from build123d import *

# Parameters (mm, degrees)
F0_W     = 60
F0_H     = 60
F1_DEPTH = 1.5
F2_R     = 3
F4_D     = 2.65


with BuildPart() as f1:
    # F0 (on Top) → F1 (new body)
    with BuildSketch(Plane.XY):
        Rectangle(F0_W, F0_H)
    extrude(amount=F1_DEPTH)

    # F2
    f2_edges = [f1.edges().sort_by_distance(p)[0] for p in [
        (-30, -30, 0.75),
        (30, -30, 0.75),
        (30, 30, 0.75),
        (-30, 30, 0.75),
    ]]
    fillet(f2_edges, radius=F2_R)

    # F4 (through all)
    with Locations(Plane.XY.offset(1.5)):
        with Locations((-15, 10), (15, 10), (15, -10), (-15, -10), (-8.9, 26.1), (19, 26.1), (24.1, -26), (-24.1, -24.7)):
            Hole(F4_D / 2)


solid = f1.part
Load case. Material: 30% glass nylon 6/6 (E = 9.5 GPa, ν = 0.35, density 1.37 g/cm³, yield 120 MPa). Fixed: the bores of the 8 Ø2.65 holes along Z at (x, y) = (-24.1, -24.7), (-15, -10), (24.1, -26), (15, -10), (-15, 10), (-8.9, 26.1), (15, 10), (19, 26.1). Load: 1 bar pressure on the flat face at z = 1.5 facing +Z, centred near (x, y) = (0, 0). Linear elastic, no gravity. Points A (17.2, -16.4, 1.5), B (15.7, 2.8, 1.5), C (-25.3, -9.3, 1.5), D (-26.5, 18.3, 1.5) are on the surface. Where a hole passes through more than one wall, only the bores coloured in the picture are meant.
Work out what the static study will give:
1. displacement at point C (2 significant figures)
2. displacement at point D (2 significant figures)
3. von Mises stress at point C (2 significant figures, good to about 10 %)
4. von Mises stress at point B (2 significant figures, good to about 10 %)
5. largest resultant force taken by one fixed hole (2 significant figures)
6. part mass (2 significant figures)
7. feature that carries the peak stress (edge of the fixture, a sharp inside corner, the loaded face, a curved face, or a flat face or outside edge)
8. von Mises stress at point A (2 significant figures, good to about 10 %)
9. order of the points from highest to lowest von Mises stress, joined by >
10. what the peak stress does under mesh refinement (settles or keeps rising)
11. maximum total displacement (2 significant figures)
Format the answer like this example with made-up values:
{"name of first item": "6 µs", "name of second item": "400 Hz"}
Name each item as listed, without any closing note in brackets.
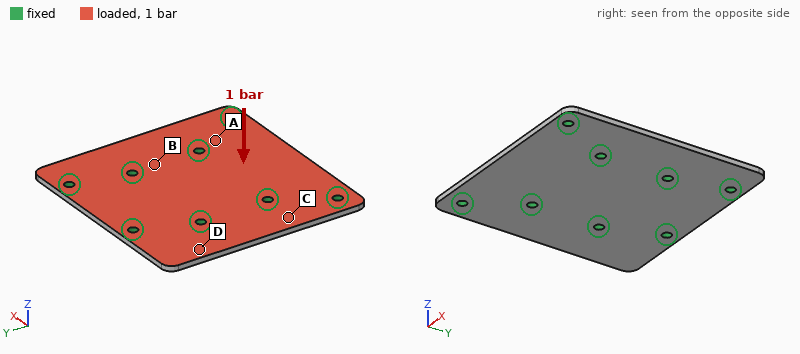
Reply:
{"displacement at point C": "0.067 mm", "displacement at point D": "0.25 mm", "von Mises stress at point C": "5.7 MPa", "von Mises stress at point B": "12 MPa", "largest resultant force taken by one fixed hole": "61 N", "part mass": "7.3 g", "feature that carries the peak stress": "edge of the fixture", "von Mises stress at point A": "16 MPa", "order of the points from highest to lowest von Mises stress, joined by >": "A > B > C > D", "what the peak stress does under mesh refinement": "keeps rising", "maximum total displacement": "0.43 mm"}
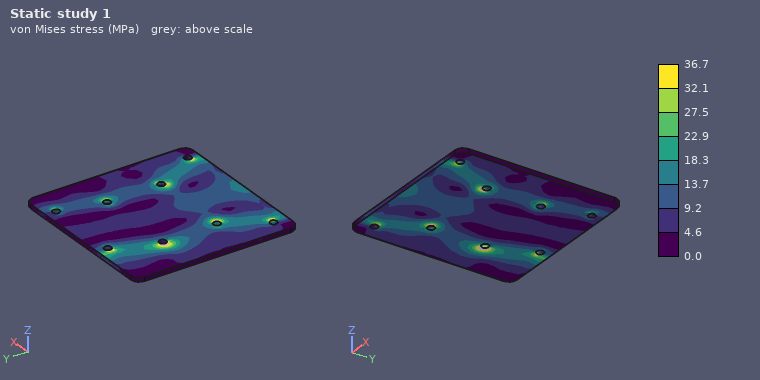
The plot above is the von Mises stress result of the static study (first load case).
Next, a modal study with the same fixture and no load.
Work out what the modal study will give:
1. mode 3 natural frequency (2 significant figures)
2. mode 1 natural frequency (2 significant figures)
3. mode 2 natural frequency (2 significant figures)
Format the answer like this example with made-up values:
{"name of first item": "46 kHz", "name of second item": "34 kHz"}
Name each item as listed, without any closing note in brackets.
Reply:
{"mode 3 natural frequency": "3400 Hz", "mode 1 natural frequency": "2300 Hz", "mode 2 natural frequency": "2500 Hz"}
